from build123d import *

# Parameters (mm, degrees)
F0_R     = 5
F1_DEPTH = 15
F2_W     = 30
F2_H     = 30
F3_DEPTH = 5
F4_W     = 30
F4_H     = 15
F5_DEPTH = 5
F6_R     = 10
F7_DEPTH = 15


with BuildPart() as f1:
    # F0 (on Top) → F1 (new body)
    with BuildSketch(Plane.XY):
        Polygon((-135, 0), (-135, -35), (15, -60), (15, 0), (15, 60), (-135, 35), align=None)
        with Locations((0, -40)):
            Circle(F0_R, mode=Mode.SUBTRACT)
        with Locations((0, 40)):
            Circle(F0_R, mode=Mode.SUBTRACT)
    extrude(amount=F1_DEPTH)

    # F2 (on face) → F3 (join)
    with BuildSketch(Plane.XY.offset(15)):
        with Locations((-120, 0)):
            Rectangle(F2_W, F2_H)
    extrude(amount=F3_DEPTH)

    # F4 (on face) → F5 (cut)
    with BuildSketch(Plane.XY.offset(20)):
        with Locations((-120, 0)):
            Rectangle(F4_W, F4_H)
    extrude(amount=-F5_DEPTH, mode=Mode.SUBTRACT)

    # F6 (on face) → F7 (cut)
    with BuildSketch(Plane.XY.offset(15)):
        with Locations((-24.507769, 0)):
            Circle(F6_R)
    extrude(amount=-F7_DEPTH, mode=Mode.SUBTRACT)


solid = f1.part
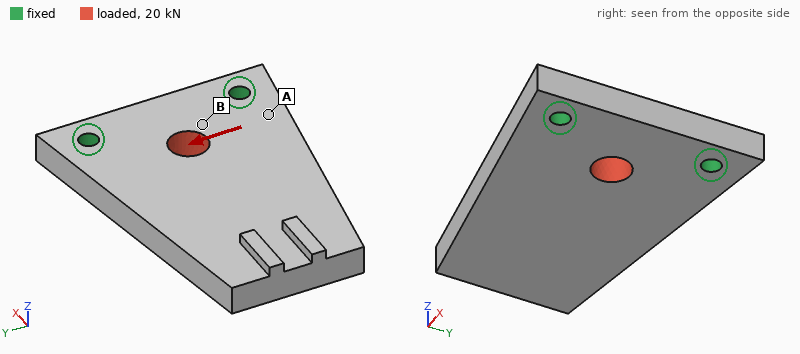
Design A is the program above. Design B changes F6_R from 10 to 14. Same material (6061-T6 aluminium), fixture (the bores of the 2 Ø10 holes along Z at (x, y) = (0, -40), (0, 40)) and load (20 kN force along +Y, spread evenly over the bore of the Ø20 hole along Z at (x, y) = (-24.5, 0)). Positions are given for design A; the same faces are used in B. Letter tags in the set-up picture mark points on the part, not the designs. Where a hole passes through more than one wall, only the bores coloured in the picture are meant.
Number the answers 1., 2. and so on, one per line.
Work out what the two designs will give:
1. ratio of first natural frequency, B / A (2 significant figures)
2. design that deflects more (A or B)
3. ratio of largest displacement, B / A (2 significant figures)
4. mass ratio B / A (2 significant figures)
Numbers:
1. 0.98
2. B
3. 1.1
4. 0.98
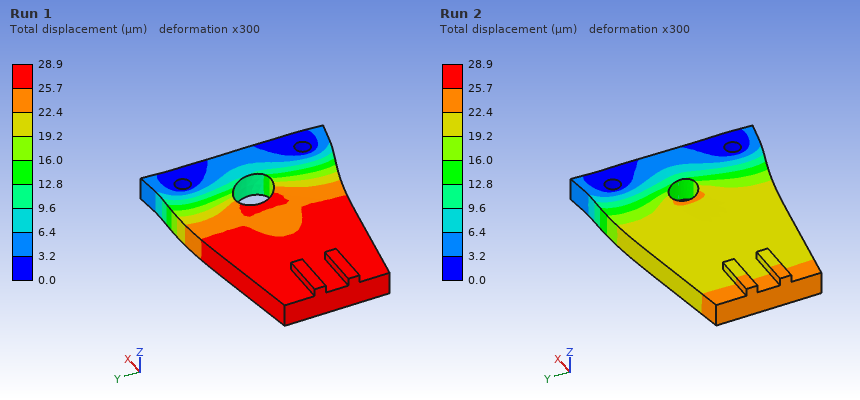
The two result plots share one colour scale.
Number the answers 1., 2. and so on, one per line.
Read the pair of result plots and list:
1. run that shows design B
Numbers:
1. Run 1
